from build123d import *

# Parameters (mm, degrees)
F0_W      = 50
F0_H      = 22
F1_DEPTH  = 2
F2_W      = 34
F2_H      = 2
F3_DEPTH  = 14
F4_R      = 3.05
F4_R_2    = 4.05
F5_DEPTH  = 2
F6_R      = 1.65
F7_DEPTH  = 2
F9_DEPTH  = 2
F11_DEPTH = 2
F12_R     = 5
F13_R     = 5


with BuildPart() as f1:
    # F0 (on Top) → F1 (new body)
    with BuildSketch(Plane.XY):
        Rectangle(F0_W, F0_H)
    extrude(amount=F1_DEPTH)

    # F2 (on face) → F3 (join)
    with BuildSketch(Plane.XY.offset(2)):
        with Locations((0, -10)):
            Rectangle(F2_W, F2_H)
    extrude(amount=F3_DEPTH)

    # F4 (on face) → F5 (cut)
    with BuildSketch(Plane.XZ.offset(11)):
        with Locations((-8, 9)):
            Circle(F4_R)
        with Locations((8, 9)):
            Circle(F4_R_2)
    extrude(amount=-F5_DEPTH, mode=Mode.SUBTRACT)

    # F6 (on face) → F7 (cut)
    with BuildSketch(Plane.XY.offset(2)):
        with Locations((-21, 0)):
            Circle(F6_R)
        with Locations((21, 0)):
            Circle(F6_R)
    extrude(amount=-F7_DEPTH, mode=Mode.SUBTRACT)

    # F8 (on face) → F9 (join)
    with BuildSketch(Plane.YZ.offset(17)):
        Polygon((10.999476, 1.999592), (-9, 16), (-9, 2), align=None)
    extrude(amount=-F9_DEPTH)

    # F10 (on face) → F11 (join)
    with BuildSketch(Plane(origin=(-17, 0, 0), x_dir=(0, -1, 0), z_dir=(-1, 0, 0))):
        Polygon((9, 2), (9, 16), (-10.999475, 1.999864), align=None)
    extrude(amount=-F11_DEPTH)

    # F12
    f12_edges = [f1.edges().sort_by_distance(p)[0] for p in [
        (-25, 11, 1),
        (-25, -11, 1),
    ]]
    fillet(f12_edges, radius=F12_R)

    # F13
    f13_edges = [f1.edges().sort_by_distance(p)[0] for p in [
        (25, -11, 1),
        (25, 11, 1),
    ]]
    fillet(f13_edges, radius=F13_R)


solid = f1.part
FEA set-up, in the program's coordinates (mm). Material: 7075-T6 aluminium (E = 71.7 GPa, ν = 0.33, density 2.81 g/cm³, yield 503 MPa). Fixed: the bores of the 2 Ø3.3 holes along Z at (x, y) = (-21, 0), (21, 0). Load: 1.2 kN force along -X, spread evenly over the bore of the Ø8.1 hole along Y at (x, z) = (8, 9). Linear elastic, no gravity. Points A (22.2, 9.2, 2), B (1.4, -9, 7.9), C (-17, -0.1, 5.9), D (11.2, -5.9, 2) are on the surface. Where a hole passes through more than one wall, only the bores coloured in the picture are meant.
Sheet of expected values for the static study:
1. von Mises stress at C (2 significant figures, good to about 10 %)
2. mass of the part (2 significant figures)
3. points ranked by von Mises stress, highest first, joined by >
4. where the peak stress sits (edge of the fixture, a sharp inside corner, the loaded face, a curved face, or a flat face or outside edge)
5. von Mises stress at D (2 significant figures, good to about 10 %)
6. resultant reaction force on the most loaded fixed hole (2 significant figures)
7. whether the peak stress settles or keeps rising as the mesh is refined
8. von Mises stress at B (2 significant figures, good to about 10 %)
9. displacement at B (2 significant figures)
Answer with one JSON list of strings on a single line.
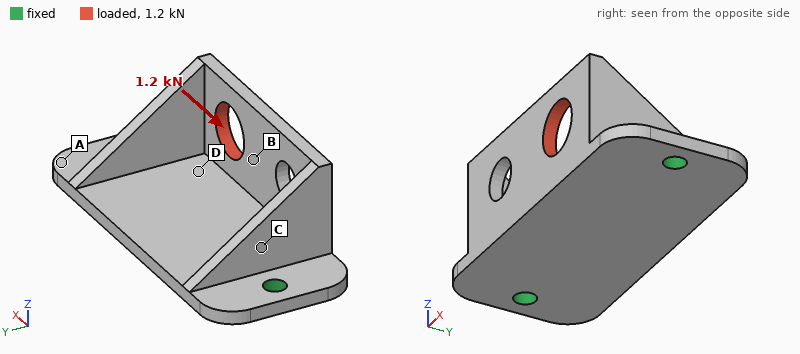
["27 MPa", "9.8 g", "B > D > C > A", "edge of the fixture", "43 MPa", "730 N", "keeps rising", "62 MPa", "31 µm"]
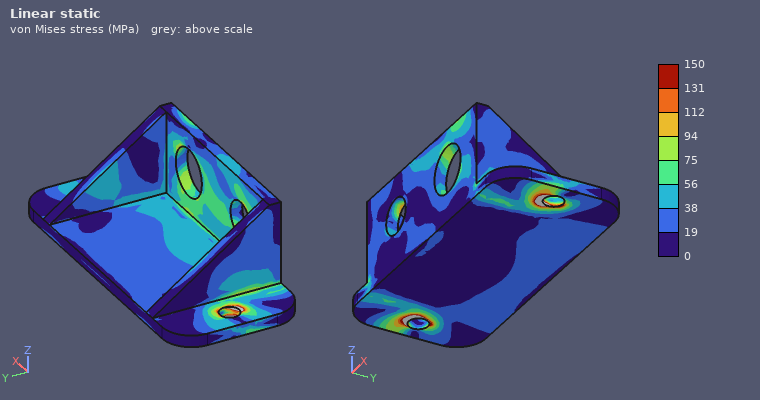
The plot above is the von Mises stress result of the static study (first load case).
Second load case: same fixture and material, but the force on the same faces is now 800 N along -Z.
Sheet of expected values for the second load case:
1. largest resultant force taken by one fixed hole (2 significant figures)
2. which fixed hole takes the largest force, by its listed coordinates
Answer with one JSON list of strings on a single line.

["600 N", "(21, 0)"]
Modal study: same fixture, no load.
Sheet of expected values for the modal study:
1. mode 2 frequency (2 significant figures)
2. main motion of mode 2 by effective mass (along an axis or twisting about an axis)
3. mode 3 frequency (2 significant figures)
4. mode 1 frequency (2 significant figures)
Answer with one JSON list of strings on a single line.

["7500 Hz", "along Z", "8600 Hz", "4800 Hz"]
